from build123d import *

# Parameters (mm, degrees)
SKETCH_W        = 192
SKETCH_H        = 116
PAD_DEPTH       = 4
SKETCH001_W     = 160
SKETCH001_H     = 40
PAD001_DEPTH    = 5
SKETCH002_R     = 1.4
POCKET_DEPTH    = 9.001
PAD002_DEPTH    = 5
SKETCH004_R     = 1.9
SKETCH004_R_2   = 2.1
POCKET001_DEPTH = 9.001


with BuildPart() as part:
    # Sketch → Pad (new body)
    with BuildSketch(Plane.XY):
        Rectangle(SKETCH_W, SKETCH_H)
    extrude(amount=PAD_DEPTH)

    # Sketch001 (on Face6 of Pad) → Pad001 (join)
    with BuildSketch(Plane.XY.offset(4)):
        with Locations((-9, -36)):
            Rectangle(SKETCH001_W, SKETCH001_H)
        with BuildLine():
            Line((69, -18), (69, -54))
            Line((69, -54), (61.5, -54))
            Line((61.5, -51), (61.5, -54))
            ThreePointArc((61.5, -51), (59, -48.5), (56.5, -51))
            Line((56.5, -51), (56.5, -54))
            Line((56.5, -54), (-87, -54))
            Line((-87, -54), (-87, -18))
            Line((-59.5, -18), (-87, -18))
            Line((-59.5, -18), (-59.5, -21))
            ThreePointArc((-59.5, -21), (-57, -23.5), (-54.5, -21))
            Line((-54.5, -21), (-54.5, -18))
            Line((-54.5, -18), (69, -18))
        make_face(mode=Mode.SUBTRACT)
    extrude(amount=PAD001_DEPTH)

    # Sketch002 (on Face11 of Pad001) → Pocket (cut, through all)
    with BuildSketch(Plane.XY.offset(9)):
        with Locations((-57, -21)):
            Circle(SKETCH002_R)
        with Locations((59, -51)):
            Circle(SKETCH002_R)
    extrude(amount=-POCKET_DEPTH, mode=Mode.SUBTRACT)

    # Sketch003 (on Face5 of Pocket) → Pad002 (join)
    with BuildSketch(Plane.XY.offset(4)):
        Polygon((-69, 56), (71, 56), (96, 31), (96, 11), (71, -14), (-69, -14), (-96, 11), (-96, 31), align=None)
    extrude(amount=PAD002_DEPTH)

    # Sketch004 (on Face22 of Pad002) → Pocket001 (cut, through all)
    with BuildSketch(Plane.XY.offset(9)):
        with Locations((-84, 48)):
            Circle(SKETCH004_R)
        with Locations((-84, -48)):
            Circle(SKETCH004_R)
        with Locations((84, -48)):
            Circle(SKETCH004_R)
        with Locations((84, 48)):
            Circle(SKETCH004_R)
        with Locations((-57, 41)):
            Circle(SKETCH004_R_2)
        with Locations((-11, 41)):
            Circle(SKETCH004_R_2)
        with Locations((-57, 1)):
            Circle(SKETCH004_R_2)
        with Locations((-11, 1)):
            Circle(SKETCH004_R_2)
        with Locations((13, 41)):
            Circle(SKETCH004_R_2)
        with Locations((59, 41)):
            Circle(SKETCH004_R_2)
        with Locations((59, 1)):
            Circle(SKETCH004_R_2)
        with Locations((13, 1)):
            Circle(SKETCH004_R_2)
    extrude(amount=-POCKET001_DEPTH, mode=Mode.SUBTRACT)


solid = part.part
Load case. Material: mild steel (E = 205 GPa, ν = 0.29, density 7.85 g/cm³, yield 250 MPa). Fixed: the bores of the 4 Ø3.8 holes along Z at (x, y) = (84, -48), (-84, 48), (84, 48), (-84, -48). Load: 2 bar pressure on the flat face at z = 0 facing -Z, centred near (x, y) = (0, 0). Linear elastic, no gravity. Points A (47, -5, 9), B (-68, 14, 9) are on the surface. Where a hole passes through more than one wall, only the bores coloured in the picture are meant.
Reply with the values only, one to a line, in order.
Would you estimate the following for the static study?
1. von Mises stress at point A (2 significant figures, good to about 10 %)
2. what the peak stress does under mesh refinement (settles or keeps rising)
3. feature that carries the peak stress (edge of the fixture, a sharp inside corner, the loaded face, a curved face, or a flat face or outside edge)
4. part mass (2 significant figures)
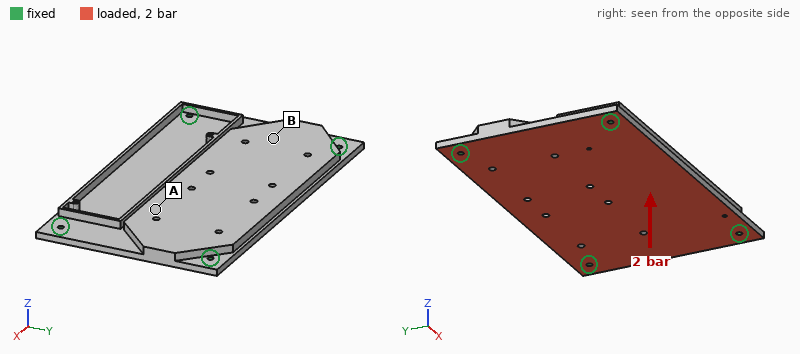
28 MPa
keeps rising
edge of the fixture
1.2 kg
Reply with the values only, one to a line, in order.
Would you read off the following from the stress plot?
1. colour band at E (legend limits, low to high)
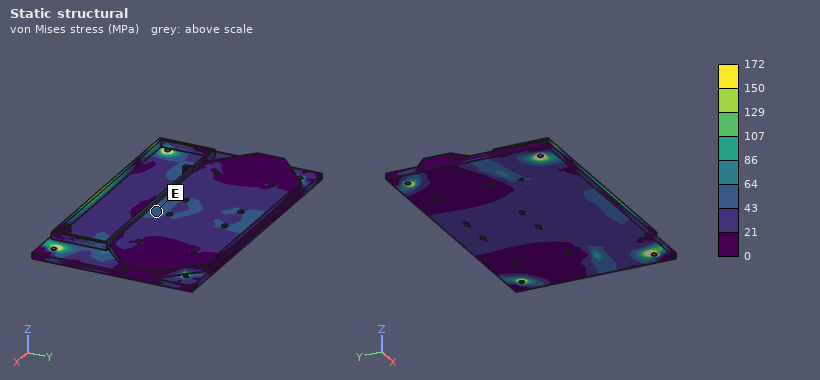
43 to 64 MPa
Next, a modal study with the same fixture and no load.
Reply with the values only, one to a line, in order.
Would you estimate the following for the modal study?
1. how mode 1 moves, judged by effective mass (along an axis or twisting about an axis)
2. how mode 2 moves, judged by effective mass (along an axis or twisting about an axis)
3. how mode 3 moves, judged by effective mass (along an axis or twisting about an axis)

along Z
twisting about X
twisting about Y
